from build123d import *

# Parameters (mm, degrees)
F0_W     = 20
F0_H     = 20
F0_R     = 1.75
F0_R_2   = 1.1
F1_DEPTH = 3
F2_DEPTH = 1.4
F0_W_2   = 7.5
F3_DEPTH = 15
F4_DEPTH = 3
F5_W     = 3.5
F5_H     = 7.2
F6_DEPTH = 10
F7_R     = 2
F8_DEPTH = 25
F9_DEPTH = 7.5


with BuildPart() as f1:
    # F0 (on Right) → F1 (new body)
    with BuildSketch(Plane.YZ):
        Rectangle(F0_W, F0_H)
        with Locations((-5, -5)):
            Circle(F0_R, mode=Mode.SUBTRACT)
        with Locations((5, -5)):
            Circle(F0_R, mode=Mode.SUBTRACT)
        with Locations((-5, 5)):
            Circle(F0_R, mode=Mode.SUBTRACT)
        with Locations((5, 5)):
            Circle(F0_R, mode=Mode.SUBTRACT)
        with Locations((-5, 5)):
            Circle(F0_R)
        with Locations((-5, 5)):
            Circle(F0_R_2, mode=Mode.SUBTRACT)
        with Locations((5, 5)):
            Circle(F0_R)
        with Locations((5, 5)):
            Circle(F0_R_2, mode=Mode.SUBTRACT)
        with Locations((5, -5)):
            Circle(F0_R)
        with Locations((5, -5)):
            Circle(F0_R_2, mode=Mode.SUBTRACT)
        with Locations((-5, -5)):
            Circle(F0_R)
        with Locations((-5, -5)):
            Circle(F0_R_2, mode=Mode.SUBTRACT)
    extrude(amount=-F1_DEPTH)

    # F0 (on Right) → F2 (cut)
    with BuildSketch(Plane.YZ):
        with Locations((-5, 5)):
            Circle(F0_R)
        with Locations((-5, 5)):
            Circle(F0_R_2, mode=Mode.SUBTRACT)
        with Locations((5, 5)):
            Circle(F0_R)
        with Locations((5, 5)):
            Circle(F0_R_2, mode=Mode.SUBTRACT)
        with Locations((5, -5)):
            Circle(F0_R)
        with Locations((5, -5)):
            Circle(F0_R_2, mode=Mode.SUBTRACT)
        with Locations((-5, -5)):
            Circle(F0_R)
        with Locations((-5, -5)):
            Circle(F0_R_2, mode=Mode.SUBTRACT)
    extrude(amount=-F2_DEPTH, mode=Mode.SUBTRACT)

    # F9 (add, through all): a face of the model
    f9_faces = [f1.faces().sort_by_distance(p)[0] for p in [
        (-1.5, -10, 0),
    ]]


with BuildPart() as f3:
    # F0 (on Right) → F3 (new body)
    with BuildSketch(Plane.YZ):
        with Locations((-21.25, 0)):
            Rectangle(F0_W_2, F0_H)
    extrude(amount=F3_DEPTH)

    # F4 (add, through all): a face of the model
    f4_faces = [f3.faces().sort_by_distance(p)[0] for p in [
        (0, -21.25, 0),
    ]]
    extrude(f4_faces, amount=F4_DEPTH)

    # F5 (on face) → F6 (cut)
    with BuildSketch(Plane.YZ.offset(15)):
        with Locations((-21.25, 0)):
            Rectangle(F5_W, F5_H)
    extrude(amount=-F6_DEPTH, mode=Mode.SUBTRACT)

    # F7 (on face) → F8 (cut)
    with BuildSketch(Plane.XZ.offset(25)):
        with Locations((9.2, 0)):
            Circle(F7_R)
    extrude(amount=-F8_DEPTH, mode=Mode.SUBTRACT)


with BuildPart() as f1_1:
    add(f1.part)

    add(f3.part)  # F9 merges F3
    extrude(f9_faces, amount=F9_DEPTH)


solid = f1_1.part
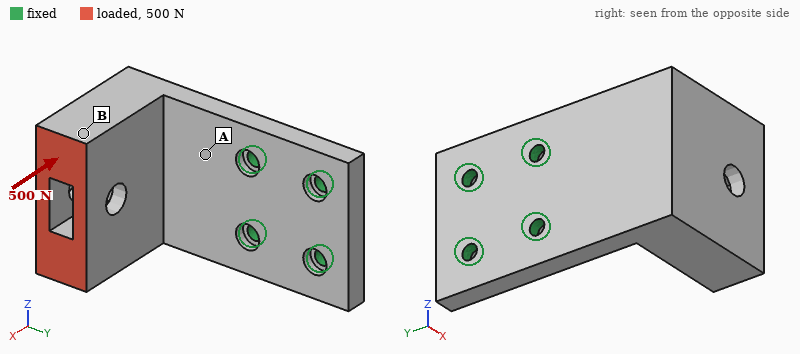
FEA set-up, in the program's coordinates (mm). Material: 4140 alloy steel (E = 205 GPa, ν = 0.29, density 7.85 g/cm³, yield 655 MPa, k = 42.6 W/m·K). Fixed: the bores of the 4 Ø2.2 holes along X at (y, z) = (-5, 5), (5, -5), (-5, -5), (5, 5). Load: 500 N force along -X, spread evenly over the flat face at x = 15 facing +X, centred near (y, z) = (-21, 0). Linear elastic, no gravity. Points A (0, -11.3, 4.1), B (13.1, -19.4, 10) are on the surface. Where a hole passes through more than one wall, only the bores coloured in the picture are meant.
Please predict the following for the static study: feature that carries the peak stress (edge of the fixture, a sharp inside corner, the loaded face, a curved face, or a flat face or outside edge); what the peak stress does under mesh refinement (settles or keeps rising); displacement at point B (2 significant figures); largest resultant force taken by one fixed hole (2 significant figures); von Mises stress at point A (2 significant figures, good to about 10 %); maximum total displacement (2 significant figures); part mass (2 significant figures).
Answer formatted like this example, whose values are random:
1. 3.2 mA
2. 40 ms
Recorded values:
1. edge of the fixture
2. keeps rising
3. 0.15 mm
4. 650 N
5. 140 MPa
6. 0.19 mm
7. 31 g
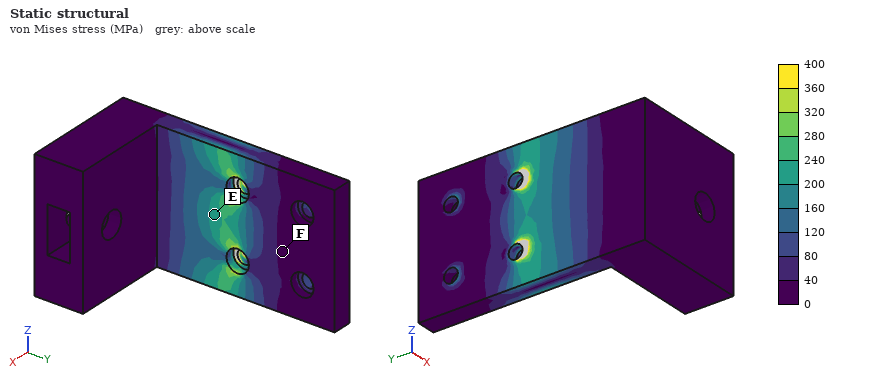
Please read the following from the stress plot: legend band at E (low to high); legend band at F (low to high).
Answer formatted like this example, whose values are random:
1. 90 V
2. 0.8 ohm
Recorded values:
1. 200 to 240 MPa
2. 0 to 40 MPa
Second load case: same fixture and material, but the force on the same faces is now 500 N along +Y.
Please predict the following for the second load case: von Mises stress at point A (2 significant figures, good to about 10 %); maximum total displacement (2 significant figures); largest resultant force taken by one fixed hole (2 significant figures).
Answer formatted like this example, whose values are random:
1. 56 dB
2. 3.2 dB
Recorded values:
1. 240 MPa
2. 0.31 mm
3. 580 N
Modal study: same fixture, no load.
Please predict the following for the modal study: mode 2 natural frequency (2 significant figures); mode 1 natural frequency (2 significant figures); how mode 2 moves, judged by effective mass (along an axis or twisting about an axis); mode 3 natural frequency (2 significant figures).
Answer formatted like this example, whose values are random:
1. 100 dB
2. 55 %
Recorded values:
1. 4300 Hz
2. 2000 Hz
3. along Z
4. 9000 Hz
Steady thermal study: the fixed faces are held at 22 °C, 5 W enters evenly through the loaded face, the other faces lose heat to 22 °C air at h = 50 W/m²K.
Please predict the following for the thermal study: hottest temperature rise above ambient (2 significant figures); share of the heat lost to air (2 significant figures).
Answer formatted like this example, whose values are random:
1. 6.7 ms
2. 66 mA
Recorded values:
1. 33 K
2. 39 %
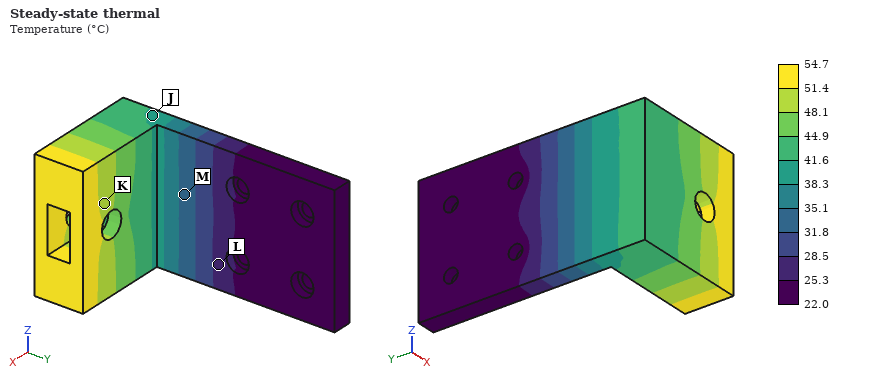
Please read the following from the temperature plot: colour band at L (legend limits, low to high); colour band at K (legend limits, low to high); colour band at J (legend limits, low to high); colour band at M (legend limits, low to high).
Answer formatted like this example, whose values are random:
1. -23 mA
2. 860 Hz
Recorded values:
1. 25.3 to 28.5 °C
2. 48.1 to 51.4 °C
3. 38.3 to 41.6 °C
4. 31.8 to 35.1 °C
